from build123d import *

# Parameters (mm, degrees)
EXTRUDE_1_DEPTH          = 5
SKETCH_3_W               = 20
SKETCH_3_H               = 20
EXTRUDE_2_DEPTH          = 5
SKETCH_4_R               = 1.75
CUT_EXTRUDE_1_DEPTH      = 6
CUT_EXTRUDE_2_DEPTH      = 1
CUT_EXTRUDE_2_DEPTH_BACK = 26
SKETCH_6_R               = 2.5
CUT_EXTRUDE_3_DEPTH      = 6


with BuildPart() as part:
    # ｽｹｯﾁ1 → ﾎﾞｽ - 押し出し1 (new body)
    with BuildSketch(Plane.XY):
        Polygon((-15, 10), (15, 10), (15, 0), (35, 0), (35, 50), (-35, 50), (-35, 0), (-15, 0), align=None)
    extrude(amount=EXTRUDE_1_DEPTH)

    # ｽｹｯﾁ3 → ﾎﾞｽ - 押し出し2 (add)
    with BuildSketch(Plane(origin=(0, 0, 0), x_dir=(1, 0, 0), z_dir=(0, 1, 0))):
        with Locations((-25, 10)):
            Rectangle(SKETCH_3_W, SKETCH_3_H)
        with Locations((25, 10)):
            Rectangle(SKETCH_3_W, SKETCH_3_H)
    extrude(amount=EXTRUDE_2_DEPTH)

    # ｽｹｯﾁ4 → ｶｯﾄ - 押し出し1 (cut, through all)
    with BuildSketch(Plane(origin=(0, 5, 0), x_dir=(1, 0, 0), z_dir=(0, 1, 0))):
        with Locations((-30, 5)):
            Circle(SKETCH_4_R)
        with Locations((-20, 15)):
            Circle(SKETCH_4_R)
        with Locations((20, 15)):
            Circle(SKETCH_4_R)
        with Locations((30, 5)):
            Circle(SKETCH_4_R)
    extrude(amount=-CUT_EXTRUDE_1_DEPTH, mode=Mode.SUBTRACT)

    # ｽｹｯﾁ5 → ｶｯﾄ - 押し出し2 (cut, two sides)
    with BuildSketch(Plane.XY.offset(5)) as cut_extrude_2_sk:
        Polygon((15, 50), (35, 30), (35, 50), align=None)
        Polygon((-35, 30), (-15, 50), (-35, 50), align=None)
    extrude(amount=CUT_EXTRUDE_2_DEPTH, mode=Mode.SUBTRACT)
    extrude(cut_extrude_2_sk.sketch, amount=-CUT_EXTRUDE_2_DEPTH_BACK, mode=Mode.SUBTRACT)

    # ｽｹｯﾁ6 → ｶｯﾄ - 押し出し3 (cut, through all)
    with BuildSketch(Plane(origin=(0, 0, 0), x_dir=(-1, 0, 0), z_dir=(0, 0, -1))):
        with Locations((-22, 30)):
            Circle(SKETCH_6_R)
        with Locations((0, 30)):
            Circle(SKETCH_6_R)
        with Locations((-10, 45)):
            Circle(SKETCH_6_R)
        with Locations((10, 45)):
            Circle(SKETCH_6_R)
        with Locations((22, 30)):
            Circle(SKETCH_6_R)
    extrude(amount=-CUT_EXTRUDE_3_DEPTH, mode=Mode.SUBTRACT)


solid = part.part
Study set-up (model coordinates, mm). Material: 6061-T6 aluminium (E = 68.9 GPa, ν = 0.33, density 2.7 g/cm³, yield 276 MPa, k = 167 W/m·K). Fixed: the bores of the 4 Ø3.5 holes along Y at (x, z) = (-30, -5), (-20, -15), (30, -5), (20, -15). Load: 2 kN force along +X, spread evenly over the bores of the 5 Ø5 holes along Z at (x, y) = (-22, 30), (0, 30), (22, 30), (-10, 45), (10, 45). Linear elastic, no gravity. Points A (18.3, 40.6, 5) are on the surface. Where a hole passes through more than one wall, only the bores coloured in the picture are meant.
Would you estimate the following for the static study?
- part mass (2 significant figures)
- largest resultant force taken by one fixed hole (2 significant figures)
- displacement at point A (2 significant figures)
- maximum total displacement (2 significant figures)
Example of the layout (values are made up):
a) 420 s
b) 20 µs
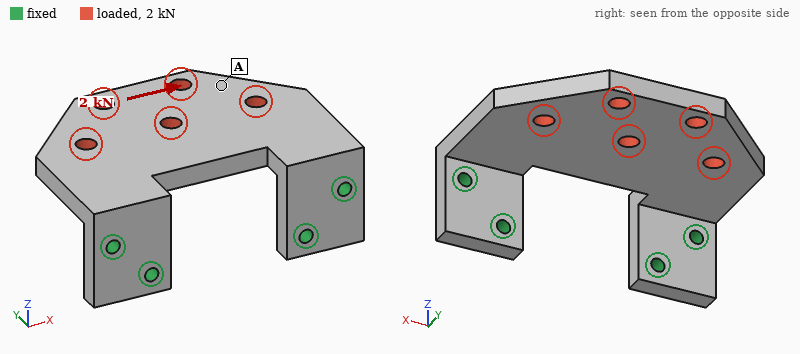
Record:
a) 47 g
b) 1.6 kN
c) 43 µm
d) 53 µm
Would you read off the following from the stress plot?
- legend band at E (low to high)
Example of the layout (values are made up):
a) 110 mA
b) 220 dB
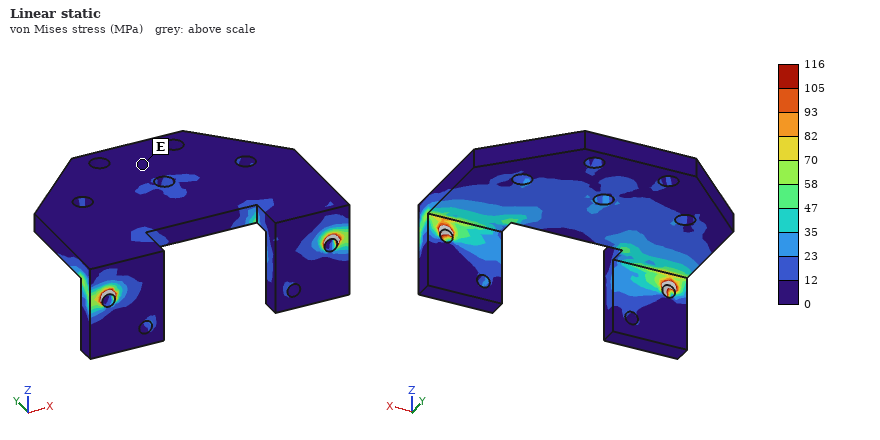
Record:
a) 0 to 12 MPa
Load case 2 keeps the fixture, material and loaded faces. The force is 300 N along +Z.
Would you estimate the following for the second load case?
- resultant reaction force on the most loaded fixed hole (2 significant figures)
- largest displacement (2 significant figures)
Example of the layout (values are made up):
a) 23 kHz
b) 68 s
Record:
a) 240 N
b) 0.31 mm
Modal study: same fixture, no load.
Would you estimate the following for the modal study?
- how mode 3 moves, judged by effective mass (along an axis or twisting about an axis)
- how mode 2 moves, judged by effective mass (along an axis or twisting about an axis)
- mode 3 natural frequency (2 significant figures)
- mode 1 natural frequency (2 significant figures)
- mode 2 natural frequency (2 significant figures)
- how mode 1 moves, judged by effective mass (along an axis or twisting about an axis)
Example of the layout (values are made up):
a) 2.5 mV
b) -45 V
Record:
a) along Y
b) twisting about Y
c) 7400 Hz
d) 1400 Hz
e) 4000 Hz
f) along Z
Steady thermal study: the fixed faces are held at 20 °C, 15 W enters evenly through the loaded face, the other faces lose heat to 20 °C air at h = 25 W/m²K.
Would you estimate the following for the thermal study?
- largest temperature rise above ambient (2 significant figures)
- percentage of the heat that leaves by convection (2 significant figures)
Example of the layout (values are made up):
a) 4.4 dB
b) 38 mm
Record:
a) 16 K
b) 11 %
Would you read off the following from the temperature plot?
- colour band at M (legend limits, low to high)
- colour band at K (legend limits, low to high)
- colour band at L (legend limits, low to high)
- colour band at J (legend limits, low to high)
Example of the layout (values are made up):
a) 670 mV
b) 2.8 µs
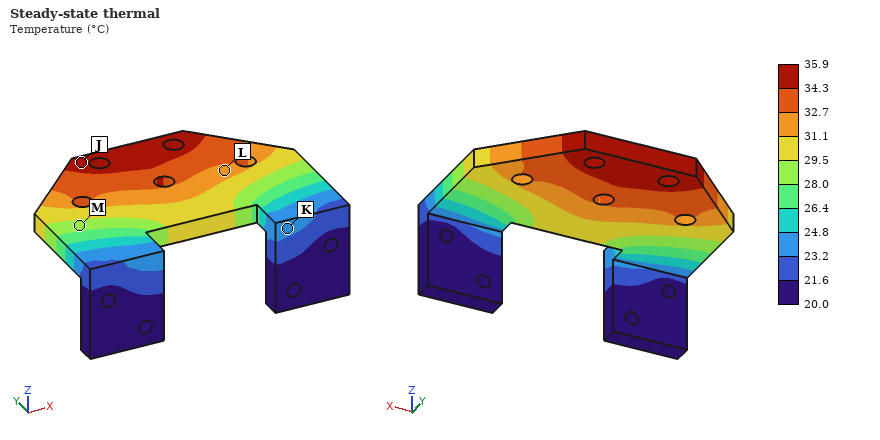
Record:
a) 28.0 to 29.5 °C
b) 23.2 to 24.8 °C
c) 31.1 to 32.7 °C
d) 34.3 to 35.9 °C
